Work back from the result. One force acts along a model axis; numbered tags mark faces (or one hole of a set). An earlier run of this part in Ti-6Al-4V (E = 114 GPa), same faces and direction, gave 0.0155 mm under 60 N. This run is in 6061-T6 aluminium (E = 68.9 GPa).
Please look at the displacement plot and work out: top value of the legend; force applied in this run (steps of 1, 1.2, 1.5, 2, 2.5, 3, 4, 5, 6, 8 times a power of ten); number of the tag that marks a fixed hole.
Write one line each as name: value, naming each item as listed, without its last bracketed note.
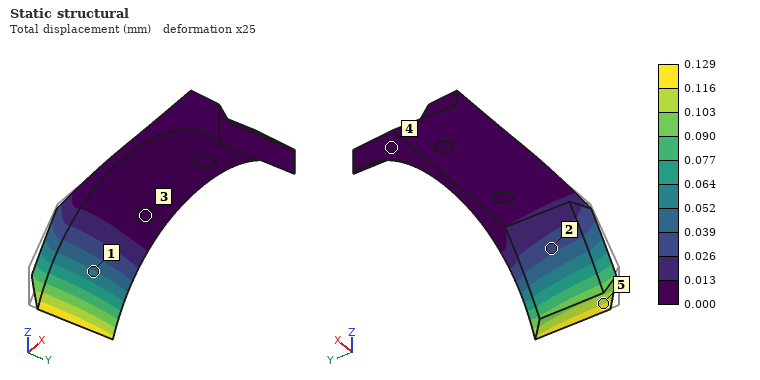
top value of the legend: 0.129 mm
force applied in this run: 300 N
number of the tag that marks a fixed hole: 3
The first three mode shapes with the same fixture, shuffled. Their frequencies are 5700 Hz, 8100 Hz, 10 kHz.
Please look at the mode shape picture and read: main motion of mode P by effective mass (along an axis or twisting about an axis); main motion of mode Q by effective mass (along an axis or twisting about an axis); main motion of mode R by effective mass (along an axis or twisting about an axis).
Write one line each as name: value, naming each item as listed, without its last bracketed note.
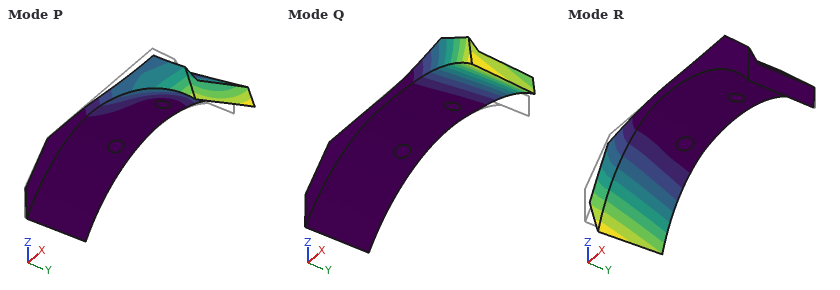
main motion of mode P by effective mass: along Y
main motion of mode Q by effective mass: along Z
main motion of mode R by effective mass: along Z
